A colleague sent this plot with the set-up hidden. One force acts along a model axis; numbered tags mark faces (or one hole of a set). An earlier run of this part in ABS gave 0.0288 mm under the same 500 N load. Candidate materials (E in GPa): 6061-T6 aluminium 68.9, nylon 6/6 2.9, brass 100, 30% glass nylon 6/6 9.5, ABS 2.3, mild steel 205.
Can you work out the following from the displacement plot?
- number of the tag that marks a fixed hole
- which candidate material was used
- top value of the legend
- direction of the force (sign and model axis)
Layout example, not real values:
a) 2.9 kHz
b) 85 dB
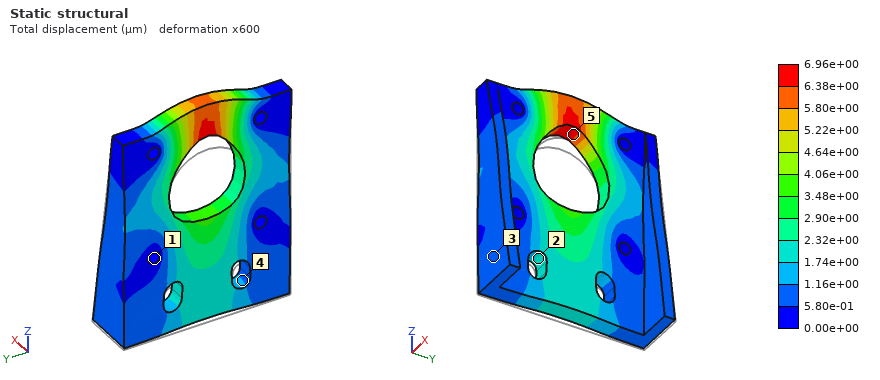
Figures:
a) 1
b) 30% glass nylon 6/6
c) 6.96e+00 µm
d) +Z
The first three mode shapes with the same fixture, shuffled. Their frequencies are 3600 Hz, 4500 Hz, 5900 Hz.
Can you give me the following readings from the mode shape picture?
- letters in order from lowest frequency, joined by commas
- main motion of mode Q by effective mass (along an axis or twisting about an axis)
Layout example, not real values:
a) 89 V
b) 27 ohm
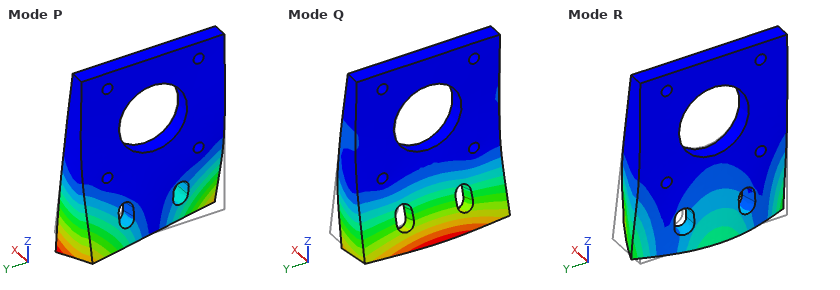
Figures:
a) Q, P, R
b) along X
